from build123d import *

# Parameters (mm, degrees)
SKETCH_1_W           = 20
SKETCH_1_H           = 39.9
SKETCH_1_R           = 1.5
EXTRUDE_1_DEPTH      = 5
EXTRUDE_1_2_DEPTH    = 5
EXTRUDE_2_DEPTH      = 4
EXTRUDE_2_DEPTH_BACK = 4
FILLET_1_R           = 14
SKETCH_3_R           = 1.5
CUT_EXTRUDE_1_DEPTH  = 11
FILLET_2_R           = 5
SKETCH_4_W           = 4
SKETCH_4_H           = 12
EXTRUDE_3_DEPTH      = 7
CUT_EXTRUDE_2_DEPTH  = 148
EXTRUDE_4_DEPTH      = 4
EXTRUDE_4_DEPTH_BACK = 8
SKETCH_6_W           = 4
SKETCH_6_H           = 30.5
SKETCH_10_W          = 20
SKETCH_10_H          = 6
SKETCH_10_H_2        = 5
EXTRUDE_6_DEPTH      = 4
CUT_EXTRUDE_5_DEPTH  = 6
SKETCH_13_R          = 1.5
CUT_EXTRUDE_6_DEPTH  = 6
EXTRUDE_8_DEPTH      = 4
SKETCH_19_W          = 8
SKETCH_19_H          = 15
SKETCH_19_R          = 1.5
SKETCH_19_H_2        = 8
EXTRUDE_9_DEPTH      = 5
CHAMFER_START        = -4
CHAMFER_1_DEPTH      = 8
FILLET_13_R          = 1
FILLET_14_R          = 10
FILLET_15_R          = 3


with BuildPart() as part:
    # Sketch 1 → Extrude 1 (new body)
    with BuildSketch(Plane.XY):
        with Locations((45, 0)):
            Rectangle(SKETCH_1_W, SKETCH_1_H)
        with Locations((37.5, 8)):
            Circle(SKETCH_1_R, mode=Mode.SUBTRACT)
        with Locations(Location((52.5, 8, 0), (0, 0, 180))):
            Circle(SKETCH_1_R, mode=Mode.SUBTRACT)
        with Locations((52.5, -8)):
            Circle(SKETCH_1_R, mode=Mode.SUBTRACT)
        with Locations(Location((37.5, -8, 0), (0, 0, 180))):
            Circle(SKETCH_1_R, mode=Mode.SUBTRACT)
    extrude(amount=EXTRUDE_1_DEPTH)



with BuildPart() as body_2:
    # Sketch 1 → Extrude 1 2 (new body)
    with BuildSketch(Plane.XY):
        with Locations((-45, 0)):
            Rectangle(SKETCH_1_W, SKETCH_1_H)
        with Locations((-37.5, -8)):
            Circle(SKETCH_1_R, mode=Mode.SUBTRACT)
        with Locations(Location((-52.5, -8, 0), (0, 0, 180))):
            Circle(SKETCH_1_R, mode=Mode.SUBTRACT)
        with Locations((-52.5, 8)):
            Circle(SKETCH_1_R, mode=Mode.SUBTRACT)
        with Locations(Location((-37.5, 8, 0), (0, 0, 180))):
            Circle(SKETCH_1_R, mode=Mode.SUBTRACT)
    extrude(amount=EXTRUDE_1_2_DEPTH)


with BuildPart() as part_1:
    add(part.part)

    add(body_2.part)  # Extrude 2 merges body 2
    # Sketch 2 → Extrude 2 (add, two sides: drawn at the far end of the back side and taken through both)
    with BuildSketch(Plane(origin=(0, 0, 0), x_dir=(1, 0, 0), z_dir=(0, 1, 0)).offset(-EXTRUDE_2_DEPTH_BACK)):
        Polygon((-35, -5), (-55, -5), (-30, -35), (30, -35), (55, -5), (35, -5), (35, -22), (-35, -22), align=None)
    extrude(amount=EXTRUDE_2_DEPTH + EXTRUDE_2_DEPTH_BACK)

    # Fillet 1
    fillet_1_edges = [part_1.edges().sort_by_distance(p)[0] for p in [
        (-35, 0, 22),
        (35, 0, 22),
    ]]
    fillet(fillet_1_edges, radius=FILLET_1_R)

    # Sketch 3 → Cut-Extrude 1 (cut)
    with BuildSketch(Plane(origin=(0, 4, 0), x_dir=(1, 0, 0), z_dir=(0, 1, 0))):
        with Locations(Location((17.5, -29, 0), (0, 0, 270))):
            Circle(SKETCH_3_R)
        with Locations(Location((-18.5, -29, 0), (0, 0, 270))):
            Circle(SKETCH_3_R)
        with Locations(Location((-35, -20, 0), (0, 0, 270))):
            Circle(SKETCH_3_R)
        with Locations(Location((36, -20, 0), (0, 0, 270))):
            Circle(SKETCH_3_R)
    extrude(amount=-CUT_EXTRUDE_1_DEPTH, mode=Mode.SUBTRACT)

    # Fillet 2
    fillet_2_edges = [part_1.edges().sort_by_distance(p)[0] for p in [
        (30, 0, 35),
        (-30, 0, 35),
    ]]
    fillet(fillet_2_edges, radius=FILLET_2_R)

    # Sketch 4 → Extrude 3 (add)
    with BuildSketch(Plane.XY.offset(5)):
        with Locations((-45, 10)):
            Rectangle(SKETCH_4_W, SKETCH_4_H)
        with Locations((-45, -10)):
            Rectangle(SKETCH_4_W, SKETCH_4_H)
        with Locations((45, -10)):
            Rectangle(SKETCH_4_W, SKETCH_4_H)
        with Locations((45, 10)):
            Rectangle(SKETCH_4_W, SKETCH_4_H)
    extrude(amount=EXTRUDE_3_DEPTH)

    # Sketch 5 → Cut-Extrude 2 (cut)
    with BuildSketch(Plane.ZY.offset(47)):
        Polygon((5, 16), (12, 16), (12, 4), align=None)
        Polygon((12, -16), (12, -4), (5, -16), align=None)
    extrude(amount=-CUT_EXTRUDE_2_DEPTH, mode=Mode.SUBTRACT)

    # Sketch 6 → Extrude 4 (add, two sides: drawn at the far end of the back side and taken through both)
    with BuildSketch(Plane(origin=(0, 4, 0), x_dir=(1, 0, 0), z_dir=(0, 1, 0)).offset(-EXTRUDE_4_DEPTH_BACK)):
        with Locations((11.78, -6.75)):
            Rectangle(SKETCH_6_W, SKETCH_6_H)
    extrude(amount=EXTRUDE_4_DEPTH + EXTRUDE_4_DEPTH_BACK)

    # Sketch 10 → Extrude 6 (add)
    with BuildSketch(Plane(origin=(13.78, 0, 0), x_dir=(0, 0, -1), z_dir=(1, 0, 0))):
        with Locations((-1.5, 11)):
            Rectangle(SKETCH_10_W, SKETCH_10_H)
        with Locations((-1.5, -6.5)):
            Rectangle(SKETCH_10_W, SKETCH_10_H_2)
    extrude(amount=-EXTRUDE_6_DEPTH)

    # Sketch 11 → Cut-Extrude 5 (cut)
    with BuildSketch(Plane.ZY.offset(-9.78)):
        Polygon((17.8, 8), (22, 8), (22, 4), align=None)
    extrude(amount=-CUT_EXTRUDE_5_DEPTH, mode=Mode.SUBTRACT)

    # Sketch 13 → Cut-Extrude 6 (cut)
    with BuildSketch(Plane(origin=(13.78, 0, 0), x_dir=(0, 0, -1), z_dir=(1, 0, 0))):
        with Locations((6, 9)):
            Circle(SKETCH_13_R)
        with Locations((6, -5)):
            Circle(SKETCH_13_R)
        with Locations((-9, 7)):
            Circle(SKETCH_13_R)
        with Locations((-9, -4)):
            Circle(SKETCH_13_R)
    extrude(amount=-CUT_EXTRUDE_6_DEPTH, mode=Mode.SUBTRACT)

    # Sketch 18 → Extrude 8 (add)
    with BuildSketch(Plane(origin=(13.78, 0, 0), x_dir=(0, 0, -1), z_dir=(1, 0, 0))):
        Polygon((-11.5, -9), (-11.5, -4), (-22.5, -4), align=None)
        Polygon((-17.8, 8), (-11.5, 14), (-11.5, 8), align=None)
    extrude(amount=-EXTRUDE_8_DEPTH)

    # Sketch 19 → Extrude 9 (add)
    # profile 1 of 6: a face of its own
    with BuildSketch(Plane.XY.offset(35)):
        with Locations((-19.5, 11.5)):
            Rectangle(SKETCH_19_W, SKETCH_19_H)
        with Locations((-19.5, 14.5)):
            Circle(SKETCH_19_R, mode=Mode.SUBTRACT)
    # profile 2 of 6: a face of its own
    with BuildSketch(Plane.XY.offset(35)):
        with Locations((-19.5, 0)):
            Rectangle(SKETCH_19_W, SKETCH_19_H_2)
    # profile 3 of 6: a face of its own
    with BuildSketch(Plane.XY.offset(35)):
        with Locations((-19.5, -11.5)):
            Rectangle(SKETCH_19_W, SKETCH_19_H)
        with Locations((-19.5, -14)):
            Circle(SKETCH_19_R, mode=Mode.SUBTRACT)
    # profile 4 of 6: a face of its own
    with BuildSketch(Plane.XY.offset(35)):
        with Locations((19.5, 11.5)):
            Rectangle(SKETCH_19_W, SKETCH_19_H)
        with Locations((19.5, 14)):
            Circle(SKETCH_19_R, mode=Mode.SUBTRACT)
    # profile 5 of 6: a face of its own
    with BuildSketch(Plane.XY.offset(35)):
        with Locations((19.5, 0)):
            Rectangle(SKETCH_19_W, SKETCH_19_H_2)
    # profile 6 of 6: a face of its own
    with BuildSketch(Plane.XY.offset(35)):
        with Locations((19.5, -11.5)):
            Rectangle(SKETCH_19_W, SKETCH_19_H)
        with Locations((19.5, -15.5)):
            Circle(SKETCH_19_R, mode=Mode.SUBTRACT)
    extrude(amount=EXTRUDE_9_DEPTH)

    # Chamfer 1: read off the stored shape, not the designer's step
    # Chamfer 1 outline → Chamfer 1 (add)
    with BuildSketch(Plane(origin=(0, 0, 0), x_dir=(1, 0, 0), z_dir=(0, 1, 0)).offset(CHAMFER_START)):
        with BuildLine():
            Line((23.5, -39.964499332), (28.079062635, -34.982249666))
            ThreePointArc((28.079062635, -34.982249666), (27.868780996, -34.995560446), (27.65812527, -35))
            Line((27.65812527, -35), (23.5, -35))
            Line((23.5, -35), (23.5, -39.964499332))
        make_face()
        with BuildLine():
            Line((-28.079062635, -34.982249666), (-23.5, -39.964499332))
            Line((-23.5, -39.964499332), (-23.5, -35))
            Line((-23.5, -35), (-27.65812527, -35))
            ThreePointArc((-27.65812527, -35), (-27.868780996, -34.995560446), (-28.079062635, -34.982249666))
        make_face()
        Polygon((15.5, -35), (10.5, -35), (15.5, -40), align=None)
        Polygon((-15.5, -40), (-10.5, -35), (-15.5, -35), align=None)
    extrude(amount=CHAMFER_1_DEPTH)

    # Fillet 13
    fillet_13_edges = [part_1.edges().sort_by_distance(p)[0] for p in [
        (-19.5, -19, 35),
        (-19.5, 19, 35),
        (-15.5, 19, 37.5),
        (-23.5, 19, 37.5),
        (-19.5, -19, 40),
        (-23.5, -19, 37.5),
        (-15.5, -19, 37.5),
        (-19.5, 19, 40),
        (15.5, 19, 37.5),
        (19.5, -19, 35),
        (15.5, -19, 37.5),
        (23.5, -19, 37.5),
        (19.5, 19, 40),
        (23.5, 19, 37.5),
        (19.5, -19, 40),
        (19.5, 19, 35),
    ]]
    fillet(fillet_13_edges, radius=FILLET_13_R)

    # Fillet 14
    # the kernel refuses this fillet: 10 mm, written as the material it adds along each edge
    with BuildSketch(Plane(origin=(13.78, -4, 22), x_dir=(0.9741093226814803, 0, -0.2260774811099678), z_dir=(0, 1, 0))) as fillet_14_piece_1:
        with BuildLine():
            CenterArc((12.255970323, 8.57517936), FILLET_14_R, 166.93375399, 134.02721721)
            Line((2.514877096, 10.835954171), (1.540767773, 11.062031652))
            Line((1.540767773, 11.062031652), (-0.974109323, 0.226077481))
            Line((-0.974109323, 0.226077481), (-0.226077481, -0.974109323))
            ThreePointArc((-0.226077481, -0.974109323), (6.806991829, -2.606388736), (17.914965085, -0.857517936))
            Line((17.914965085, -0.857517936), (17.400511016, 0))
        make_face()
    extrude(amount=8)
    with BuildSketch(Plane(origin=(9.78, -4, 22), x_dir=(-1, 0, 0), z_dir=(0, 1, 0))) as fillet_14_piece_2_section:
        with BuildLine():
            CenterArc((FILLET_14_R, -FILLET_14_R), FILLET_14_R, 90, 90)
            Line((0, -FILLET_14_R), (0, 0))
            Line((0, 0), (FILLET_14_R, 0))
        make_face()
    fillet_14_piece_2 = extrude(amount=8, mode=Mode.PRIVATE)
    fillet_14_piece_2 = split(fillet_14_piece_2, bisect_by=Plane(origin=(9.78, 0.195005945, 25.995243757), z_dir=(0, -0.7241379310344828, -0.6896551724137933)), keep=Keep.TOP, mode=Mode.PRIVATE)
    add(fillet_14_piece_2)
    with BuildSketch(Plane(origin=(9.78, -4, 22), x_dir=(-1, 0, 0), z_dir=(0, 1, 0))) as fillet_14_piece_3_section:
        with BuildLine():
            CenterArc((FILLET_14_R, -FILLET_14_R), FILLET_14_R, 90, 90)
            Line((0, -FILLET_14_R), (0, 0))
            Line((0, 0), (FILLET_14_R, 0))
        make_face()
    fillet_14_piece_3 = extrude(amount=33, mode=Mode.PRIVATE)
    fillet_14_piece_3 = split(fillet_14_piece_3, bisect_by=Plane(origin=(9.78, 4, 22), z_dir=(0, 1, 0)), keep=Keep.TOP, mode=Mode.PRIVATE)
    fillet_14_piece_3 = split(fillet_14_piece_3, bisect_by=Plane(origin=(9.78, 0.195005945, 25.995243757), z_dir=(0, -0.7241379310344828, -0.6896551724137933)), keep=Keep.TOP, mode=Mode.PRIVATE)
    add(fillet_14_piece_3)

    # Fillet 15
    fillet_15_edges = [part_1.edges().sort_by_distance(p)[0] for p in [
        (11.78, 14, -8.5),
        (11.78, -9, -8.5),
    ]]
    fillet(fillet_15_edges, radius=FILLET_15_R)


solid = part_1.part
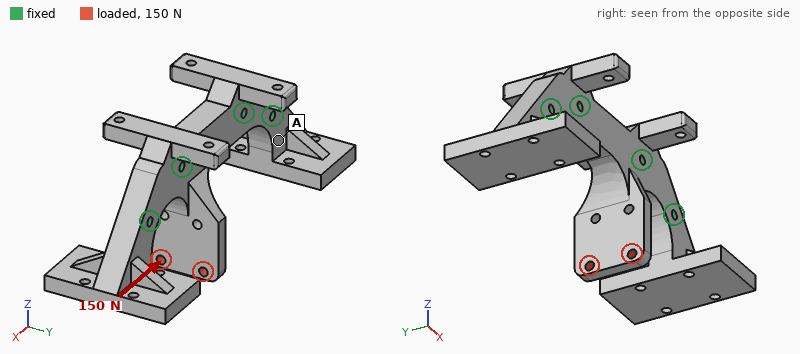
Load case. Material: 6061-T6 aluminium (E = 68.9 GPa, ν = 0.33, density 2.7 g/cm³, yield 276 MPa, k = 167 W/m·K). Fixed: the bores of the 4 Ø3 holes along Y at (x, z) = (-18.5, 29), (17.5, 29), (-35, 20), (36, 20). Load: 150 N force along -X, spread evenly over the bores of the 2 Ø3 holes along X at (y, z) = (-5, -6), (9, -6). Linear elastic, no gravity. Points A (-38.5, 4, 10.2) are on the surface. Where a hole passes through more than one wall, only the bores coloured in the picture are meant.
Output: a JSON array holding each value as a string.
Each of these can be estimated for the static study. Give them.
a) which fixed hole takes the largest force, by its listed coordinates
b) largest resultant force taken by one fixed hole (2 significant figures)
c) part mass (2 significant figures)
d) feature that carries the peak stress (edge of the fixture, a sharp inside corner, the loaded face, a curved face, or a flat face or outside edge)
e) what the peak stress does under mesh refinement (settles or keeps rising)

["(-18.5, 29)", "160 N", "70 g", "a sharp inside corner", "keeps rising"]
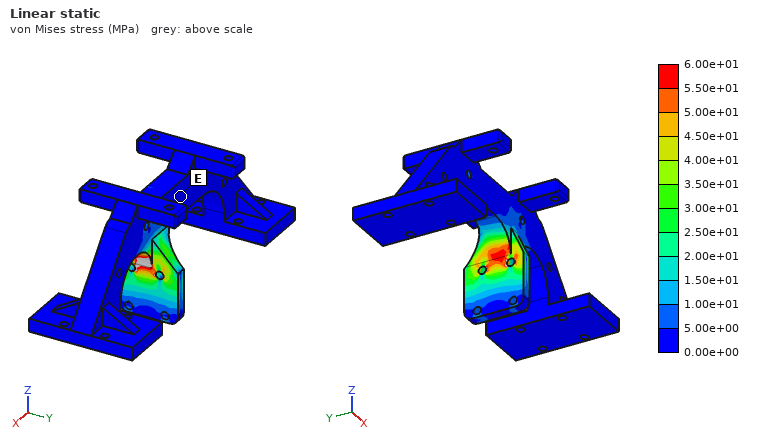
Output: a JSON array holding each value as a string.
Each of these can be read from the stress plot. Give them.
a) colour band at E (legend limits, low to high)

["0.00e+00 to 5.00e+00 MPa"]
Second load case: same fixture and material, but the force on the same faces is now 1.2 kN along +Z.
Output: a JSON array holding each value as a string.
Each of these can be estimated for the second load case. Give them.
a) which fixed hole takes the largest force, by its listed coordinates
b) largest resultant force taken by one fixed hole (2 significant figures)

["(17.5, 29)", "1.1 kN"]
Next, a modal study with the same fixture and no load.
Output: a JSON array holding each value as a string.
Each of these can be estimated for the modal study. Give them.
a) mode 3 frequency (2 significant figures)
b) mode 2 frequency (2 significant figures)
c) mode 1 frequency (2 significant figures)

["4400 Hz", "3900 Hz", "3800 Hz"]
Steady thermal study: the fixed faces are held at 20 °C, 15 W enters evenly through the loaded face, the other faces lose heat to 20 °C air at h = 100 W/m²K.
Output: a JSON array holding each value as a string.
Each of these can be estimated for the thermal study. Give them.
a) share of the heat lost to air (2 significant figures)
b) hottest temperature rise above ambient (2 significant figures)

["24 %", "34 K"]
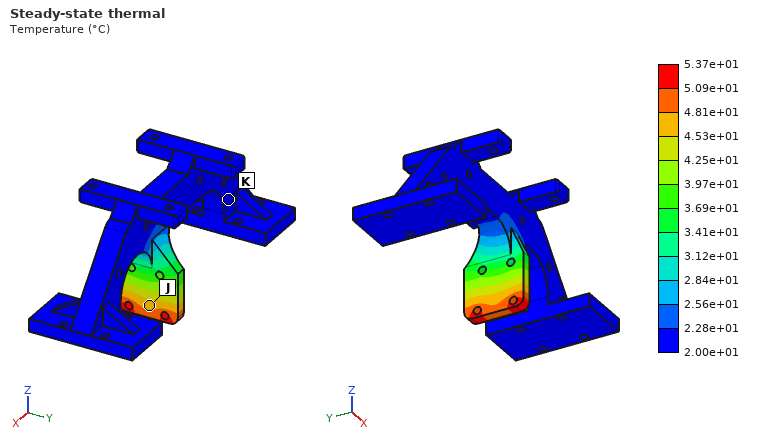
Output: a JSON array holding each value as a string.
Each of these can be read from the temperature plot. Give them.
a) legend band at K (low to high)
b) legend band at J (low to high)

["2.00e+01 to 2.28e+01 °C", "4.53e+01 to 4.81e+01 °C"]
